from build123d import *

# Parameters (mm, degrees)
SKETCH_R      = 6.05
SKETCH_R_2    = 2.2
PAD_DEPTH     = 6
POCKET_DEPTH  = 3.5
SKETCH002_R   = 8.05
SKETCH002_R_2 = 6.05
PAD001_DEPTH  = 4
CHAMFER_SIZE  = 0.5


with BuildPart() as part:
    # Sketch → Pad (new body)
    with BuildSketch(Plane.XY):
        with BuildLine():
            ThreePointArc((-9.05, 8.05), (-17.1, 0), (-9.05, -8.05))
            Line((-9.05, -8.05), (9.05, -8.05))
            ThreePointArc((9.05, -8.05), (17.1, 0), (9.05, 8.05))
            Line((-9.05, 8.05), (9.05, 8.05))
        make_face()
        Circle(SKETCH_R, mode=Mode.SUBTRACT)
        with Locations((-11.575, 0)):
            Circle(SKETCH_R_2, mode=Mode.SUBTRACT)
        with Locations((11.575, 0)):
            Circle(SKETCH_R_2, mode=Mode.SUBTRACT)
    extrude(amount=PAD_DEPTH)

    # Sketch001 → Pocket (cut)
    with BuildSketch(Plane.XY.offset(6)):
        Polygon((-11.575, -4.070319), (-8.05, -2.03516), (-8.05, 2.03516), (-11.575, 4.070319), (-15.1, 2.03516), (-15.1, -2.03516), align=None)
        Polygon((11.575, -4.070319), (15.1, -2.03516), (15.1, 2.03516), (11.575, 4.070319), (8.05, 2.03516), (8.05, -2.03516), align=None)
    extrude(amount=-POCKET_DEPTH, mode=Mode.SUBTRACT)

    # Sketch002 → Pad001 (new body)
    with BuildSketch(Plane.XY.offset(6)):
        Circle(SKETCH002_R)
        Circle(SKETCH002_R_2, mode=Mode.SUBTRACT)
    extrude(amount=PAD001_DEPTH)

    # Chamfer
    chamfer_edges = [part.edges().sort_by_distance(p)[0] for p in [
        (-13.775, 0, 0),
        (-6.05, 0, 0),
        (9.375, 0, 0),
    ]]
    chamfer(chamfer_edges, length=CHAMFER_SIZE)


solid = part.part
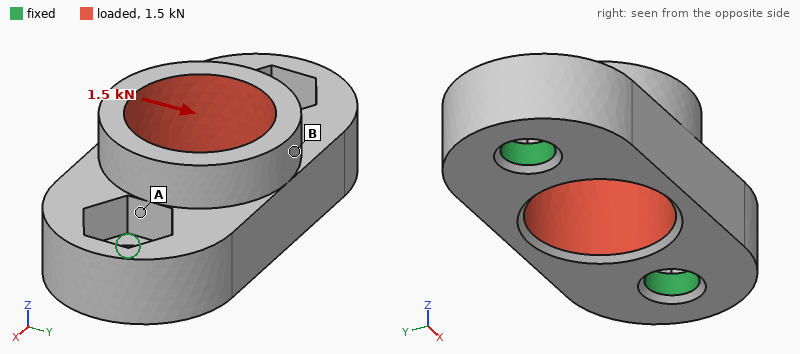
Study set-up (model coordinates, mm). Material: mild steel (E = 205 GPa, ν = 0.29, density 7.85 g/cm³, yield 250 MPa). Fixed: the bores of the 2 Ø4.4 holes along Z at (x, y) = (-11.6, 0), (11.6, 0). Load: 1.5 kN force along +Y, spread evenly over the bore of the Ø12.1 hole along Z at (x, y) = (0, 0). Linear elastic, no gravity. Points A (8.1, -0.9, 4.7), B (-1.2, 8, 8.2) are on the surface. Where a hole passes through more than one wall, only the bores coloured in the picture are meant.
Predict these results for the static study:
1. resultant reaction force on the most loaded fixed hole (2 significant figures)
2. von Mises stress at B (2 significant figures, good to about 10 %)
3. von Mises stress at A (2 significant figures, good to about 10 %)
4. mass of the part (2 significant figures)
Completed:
750 N
23 MPa
53 MPa
18 g
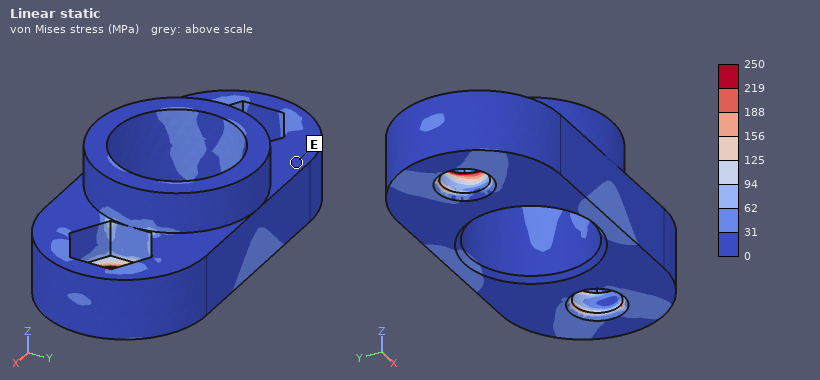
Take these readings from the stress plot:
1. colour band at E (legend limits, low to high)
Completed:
0 to 31 MPa
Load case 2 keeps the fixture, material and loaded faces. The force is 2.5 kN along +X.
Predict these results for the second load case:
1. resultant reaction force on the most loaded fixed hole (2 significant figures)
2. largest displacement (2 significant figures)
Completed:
1.3 kN
3.7 µm
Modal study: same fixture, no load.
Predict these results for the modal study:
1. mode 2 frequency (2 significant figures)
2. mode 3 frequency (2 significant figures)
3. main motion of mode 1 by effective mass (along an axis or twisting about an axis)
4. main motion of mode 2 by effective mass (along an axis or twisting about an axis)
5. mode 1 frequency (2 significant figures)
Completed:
29 kHz
35 kHz
along Y
along Z
17 kHz
